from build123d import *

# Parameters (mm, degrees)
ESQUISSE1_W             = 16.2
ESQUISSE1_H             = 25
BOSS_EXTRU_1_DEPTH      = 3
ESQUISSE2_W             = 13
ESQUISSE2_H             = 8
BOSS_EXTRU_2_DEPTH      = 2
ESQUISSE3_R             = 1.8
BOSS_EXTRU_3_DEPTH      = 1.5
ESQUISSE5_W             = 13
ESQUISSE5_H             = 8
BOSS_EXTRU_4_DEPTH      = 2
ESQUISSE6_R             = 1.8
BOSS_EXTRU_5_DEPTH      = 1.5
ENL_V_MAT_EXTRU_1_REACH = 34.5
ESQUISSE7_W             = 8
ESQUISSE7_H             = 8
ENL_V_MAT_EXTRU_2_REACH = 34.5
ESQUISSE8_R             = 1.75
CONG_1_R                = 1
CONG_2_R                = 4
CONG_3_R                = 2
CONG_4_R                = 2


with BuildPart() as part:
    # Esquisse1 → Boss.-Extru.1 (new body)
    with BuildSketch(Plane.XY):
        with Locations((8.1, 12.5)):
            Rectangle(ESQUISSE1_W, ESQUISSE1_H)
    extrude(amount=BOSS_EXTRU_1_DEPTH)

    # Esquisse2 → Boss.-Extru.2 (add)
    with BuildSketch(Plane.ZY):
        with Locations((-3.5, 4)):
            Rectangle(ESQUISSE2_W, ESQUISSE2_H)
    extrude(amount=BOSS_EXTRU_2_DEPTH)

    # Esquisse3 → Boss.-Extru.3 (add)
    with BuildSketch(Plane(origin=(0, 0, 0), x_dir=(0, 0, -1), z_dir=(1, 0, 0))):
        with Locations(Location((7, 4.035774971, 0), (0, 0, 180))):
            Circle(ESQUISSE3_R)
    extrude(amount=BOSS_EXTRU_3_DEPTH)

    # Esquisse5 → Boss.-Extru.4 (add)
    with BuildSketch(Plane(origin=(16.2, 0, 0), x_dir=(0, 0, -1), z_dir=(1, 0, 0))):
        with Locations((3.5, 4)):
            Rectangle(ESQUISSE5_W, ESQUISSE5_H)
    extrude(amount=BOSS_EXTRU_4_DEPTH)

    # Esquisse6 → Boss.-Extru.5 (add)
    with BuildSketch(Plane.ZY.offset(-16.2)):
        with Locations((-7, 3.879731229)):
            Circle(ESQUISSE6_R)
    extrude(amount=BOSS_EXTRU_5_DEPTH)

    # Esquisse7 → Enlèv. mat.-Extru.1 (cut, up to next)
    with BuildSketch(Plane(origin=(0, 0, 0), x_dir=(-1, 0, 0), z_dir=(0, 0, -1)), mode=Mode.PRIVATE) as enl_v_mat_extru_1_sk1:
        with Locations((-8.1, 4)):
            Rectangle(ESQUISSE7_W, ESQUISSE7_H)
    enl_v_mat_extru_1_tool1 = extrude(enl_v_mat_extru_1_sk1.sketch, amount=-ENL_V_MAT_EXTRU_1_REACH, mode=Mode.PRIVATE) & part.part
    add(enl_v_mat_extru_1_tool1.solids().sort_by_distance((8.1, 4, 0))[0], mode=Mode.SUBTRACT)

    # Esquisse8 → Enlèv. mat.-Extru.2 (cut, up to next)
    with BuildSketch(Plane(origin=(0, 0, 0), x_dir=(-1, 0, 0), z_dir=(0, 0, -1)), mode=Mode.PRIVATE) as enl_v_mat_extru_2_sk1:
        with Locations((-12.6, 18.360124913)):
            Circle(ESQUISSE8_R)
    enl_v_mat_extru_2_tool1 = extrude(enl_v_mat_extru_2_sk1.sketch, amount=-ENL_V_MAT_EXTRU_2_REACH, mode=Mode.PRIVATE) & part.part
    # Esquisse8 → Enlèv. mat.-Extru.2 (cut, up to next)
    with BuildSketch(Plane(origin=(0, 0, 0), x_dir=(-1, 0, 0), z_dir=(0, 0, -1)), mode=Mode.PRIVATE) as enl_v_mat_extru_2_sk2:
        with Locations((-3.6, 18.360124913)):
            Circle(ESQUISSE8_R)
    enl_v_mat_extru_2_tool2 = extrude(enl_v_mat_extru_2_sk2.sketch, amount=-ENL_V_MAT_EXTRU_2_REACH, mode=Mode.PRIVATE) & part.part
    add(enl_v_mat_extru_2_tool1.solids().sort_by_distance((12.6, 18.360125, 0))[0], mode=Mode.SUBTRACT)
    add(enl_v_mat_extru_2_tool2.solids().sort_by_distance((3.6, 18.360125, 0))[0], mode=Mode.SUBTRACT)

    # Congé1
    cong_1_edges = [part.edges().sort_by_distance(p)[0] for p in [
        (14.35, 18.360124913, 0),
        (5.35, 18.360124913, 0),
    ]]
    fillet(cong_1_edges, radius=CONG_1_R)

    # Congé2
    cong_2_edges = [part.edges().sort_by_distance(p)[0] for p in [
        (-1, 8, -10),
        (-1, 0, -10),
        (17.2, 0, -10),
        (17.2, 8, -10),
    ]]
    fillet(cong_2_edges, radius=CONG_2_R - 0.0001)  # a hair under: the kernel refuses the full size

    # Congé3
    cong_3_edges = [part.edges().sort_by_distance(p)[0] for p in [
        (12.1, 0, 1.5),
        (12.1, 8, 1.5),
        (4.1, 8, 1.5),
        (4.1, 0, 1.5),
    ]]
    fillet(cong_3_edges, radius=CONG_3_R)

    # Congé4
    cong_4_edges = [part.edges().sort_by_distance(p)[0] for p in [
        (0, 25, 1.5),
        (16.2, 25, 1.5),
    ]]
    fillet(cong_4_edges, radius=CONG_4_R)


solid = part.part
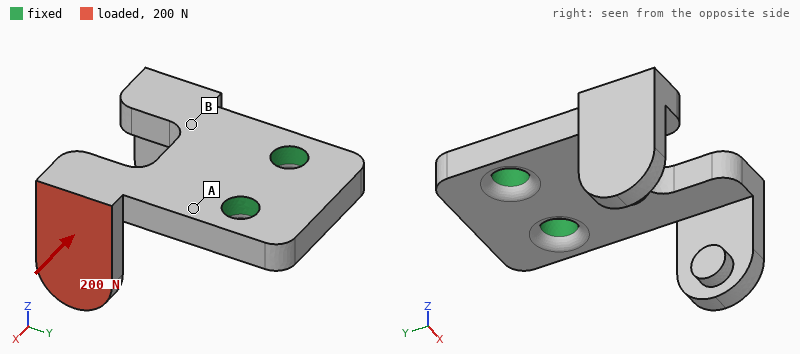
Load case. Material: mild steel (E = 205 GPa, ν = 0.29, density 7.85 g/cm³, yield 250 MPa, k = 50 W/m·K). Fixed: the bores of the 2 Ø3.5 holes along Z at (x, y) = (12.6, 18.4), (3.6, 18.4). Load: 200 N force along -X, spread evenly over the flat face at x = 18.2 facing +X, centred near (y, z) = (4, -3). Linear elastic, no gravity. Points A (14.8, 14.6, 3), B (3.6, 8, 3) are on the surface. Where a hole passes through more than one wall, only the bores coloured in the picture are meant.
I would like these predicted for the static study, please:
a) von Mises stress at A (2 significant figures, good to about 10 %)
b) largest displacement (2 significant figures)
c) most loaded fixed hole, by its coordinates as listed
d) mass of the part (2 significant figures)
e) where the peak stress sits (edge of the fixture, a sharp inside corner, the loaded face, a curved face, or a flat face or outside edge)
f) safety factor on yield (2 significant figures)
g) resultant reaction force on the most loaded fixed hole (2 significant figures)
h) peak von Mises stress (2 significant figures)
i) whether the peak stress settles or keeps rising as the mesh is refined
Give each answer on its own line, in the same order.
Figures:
62 MPa
67 µm
(3.6, 18.4)
11 g
a curved face
1.0
310 N
240 MPa
settles
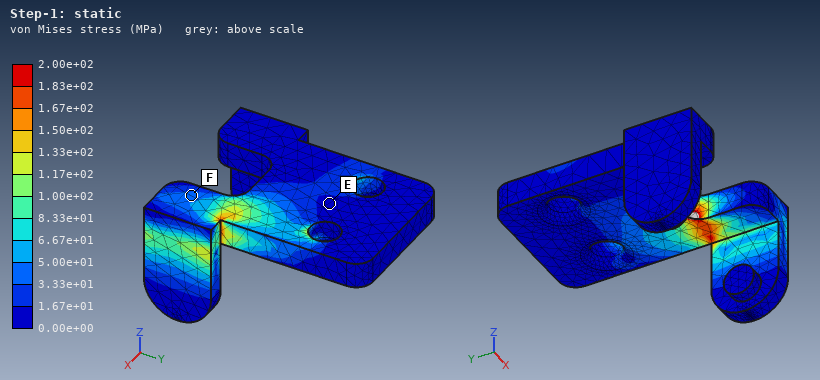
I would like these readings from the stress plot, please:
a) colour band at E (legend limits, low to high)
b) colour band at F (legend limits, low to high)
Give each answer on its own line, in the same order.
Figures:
0.00e+00 to 1.67e+01 MPa
3.33e+01 to 5.00e+01 MPa
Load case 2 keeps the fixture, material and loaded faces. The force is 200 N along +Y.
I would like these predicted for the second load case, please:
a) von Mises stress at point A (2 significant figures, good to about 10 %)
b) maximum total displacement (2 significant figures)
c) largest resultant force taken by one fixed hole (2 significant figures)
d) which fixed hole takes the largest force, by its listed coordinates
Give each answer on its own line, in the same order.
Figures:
33 MPa
56 µm
290 N
(12.6, 18.4)
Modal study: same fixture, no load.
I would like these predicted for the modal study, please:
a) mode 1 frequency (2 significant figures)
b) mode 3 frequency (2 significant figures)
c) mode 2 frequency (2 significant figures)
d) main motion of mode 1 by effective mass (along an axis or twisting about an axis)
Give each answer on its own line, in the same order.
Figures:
5000 Hz
8200 Hz
5800 Hz
along Z
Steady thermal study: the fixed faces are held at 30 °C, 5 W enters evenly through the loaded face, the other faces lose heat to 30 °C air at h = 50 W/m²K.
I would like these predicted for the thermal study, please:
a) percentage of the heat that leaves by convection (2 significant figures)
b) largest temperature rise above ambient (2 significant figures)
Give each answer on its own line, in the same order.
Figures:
21 %
75 K
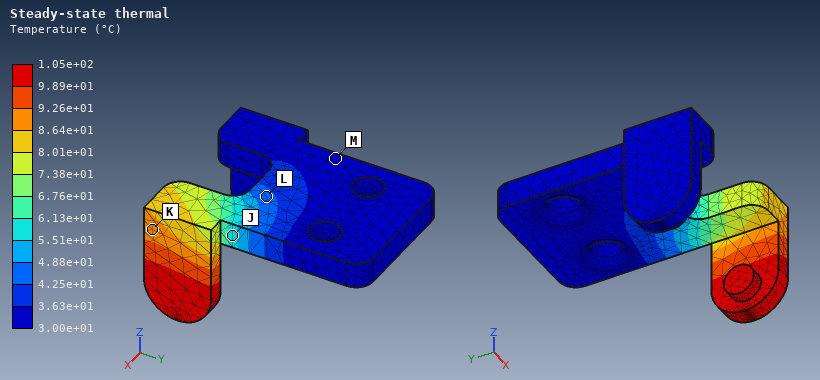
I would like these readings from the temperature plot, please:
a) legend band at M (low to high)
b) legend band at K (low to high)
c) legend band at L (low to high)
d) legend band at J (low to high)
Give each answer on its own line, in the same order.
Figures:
3.00e+01 to 3.63e+01 °C
8.64e+01 to 9.26e+01 °C
4.25e+01 to 4.88e+01 °C
5.51e+01 to 6.13e+01 °C
